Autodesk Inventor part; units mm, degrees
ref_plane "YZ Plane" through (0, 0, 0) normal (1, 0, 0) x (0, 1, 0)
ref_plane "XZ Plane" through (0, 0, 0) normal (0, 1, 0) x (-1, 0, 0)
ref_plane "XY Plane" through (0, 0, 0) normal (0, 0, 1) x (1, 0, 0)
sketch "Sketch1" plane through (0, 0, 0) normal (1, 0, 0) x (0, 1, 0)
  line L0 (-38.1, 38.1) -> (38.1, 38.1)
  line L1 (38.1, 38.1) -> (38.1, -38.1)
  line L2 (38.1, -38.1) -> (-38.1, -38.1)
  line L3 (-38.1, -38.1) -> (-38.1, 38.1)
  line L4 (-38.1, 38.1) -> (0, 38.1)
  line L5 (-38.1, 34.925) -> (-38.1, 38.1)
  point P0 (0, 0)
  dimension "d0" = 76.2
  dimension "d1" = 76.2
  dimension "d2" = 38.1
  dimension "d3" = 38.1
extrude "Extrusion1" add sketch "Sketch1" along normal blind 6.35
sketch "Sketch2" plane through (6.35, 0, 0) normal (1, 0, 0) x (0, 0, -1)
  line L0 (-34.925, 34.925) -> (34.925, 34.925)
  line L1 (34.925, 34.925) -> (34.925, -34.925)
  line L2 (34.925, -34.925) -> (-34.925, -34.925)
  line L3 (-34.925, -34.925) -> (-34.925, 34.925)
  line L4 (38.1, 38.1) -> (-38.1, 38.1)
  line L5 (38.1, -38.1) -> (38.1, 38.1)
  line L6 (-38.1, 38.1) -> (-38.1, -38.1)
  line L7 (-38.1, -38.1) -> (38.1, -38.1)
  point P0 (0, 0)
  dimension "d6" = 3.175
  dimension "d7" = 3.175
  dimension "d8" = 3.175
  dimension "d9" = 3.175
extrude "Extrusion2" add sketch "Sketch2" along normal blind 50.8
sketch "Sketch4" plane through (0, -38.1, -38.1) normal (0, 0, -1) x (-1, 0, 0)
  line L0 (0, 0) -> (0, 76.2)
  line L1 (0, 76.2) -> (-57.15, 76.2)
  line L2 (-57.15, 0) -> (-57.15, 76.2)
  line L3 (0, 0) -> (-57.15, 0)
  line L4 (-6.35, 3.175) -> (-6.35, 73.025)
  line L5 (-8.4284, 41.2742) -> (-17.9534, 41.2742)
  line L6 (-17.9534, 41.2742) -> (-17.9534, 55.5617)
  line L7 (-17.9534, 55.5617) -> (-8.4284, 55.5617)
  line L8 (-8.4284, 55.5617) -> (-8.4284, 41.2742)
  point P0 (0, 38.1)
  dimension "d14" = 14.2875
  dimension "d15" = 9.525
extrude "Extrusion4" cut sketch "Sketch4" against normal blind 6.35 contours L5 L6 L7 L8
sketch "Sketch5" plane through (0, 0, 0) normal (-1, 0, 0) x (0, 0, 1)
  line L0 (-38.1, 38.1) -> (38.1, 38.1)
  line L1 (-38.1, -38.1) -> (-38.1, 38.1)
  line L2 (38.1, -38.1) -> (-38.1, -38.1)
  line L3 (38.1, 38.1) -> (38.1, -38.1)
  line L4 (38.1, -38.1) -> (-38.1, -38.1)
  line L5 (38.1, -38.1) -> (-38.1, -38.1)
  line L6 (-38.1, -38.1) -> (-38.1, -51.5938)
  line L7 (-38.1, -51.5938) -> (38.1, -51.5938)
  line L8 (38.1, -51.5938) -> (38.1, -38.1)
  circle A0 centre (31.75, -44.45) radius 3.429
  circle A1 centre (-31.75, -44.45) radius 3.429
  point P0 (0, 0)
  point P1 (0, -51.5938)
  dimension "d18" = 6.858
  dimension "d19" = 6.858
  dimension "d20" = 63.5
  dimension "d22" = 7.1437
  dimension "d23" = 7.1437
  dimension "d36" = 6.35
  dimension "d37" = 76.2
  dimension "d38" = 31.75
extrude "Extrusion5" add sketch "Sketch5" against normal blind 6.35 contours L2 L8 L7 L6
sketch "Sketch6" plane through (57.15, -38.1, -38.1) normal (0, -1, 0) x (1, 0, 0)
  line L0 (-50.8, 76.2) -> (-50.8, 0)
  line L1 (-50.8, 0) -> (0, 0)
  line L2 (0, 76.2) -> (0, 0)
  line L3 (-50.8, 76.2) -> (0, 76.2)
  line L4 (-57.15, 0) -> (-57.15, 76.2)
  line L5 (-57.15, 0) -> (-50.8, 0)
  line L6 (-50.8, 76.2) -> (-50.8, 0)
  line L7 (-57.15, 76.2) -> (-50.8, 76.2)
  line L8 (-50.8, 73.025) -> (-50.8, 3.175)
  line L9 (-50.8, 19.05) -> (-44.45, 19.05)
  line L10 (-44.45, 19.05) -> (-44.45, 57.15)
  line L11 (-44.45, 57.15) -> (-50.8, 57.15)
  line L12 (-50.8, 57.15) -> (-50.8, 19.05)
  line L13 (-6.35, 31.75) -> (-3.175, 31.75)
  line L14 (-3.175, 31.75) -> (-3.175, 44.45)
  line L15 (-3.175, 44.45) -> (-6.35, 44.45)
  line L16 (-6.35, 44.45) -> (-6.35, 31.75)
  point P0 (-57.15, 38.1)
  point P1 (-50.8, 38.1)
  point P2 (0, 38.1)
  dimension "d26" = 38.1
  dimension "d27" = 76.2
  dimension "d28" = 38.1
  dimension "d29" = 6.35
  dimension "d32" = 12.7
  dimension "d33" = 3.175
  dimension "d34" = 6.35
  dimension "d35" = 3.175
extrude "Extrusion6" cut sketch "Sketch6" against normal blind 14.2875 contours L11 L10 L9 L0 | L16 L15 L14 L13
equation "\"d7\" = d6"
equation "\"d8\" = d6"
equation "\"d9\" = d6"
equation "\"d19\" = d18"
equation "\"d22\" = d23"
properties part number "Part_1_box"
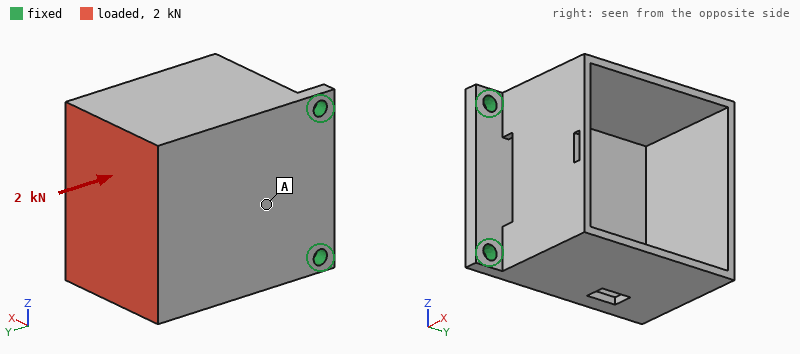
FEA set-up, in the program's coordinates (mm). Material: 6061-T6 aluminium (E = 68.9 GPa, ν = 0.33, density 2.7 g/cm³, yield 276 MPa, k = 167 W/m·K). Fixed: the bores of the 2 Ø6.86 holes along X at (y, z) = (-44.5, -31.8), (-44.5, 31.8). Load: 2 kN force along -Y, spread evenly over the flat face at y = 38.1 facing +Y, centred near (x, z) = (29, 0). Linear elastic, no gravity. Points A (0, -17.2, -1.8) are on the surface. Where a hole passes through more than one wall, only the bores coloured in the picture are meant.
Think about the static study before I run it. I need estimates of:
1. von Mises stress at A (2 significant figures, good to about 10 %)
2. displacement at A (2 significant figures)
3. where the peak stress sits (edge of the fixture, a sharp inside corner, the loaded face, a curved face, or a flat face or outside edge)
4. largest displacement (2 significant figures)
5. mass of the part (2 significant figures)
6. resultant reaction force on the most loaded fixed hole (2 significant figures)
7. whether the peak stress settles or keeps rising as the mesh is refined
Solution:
18 MPa
0.15 mm
edge of the fixture
0.97 mm
240 g
1.0 kN
keeps rising
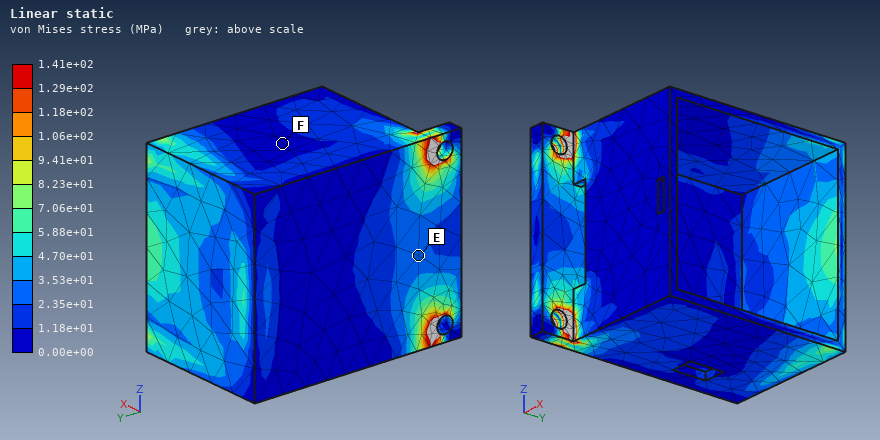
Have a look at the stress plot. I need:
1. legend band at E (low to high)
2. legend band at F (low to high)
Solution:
2.35e+01 to 3.53e+01 MPa
0.00e+00 to 1.18e+01 MPa
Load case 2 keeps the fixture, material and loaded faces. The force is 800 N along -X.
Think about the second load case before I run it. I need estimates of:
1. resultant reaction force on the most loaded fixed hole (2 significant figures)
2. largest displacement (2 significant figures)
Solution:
520 N
0.91 mm
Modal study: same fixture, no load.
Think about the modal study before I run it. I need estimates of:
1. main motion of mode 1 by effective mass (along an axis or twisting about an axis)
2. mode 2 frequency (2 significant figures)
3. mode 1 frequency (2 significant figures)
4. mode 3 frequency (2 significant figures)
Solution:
along X
970 Hz
510 Hz
2200 Hz
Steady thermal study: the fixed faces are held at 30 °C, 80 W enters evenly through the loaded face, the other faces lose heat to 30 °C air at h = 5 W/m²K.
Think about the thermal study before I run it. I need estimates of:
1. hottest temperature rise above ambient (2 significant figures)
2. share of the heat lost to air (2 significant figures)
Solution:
80 K
9.3 %
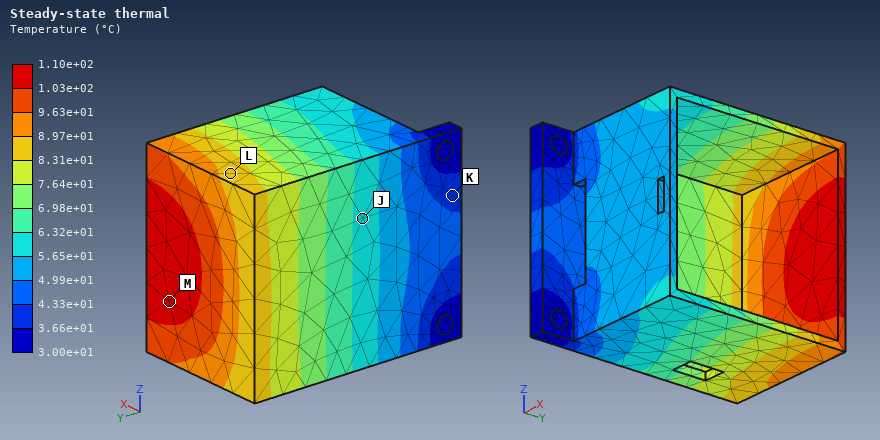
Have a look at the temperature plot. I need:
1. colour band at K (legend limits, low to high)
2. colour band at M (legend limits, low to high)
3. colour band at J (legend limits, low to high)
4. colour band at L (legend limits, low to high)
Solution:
3.66e+01 to 4.33e+01 °C
1.03e+02 to 1.10e+02 °C
5.65e+01 to 6.32e+01 °C
8.31e+01 to 8.97e+01 °C
